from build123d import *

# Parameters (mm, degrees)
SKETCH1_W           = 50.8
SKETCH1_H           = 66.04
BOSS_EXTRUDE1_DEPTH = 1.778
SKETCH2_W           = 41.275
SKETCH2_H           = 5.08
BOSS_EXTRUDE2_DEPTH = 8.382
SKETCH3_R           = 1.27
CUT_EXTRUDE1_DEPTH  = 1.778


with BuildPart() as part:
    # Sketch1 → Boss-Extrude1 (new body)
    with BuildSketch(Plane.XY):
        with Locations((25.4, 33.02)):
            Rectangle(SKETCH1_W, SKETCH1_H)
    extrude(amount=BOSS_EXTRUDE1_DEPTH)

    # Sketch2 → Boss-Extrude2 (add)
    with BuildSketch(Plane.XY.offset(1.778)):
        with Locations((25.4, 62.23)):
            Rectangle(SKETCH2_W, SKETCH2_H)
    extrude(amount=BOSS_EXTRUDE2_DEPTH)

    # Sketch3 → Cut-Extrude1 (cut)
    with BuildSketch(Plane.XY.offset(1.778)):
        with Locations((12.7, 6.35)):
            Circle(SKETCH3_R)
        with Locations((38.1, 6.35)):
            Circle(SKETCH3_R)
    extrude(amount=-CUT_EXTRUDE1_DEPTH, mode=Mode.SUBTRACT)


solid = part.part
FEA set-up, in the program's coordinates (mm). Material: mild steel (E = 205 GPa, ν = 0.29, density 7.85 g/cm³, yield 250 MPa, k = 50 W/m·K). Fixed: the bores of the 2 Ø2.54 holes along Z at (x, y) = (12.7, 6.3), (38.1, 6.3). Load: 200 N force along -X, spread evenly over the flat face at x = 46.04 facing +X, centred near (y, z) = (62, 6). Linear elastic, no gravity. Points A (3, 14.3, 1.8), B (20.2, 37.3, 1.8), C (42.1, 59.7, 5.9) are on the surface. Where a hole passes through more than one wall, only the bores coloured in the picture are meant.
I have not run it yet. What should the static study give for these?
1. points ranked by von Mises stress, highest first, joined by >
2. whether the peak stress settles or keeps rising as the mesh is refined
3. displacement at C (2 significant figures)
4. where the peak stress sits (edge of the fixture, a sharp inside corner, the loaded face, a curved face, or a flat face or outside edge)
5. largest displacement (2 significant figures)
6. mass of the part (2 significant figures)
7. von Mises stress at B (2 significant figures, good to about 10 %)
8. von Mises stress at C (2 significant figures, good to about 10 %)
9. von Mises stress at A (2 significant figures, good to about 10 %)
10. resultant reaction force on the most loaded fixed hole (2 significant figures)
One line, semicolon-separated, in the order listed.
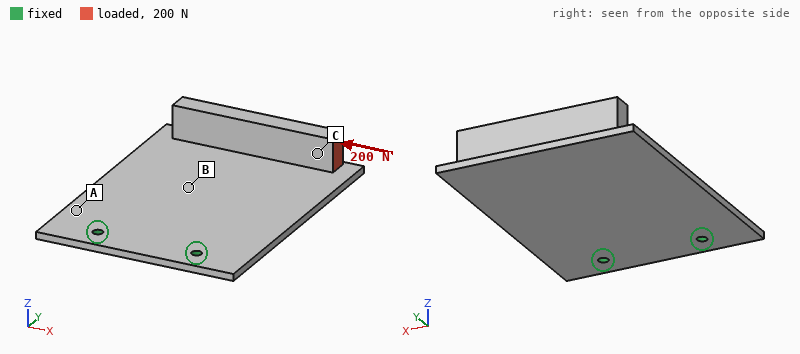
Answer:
B > A > C; keeps rising; 0.086 mm; edge of the fixture; 0.12 mm; 60 g; 34 MPa; 7.8 MPa; 17 MPa; 430 N
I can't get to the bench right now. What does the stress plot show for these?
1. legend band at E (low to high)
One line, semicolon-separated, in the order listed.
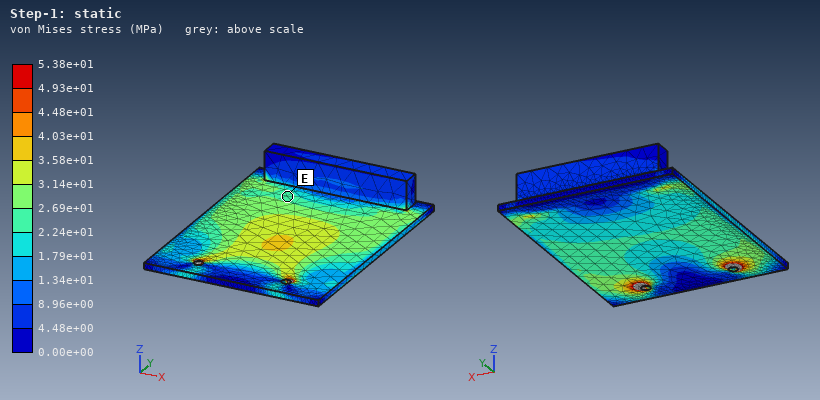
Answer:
2.24e+01 to 2.69e+01 MPa
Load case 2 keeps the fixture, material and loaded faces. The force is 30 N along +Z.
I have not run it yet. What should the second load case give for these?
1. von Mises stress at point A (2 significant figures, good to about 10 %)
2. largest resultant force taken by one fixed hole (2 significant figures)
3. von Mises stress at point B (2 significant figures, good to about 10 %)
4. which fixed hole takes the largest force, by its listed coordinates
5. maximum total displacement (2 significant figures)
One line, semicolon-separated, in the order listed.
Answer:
42 MPa; 34 N; 31 MPa; (38.1, 6.3); 0.49 mm
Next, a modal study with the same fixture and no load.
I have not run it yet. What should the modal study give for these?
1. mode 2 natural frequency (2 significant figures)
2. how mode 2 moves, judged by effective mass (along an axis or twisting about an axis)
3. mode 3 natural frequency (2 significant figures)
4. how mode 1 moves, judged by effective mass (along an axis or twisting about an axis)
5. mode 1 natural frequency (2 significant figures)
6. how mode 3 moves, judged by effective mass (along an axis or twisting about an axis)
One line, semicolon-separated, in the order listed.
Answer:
920 Hz; twisting about Y; 2000 Hz; along Z; 270 Hz; along Z
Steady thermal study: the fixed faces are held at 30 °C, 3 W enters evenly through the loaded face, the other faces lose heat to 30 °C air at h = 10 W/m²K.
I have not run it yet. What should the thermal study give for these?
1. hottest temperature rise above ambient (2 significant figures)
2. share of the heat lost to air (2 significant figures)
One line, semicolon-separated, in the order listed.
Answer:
42 K; 40 %
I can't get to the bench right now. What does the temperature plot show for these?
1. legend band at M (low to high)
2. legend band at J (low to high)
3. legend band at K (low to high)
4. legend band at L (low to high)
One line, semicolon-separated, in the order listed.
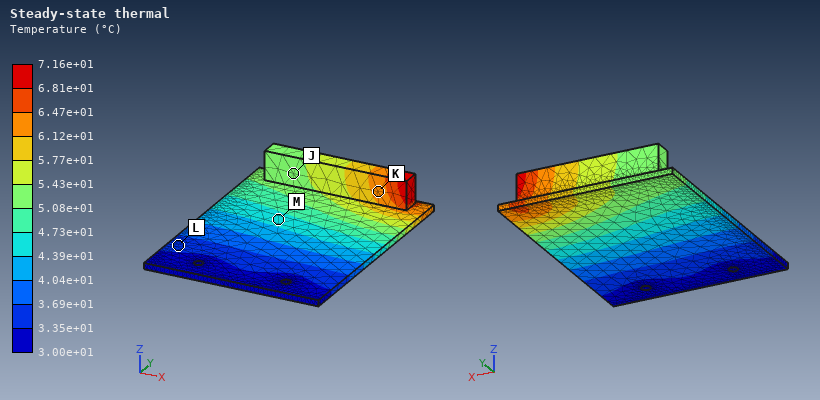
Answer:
4.39e+01 to 4.73e+01 °C; 5.08e+01 to 5.43e+01 °C; 6.12e+01 to 6.47e+01 °C; 3.35e+01 to 3.69e+01 °C
